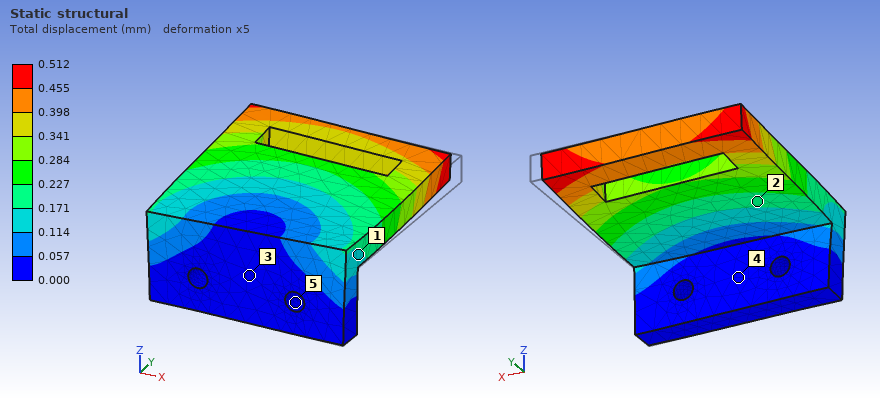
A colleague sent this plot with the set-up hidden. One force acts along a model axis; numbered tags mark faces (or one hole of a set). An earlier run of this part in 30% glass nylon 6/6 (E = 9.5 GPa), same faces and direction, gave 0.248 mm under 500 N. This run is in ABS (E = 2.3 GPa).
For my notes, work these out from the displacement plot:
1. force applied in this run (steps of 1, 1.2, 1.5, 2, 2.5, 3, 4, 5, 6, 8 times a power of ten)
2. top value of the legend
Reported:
250 N
0.512 mm
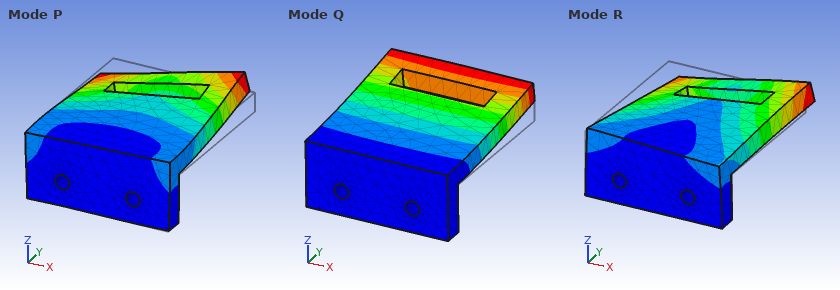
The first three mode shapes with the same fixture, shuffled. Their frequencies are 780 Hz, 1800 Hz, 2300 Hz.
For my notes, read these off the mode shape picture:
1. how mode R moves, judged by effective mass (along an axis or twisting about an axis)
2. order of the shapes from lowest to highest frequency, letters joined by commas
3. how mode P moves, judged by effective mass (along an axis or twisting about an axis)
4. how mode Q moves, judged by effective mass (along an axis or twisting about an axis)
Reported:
along X
Q, R, P
along X
along Z
